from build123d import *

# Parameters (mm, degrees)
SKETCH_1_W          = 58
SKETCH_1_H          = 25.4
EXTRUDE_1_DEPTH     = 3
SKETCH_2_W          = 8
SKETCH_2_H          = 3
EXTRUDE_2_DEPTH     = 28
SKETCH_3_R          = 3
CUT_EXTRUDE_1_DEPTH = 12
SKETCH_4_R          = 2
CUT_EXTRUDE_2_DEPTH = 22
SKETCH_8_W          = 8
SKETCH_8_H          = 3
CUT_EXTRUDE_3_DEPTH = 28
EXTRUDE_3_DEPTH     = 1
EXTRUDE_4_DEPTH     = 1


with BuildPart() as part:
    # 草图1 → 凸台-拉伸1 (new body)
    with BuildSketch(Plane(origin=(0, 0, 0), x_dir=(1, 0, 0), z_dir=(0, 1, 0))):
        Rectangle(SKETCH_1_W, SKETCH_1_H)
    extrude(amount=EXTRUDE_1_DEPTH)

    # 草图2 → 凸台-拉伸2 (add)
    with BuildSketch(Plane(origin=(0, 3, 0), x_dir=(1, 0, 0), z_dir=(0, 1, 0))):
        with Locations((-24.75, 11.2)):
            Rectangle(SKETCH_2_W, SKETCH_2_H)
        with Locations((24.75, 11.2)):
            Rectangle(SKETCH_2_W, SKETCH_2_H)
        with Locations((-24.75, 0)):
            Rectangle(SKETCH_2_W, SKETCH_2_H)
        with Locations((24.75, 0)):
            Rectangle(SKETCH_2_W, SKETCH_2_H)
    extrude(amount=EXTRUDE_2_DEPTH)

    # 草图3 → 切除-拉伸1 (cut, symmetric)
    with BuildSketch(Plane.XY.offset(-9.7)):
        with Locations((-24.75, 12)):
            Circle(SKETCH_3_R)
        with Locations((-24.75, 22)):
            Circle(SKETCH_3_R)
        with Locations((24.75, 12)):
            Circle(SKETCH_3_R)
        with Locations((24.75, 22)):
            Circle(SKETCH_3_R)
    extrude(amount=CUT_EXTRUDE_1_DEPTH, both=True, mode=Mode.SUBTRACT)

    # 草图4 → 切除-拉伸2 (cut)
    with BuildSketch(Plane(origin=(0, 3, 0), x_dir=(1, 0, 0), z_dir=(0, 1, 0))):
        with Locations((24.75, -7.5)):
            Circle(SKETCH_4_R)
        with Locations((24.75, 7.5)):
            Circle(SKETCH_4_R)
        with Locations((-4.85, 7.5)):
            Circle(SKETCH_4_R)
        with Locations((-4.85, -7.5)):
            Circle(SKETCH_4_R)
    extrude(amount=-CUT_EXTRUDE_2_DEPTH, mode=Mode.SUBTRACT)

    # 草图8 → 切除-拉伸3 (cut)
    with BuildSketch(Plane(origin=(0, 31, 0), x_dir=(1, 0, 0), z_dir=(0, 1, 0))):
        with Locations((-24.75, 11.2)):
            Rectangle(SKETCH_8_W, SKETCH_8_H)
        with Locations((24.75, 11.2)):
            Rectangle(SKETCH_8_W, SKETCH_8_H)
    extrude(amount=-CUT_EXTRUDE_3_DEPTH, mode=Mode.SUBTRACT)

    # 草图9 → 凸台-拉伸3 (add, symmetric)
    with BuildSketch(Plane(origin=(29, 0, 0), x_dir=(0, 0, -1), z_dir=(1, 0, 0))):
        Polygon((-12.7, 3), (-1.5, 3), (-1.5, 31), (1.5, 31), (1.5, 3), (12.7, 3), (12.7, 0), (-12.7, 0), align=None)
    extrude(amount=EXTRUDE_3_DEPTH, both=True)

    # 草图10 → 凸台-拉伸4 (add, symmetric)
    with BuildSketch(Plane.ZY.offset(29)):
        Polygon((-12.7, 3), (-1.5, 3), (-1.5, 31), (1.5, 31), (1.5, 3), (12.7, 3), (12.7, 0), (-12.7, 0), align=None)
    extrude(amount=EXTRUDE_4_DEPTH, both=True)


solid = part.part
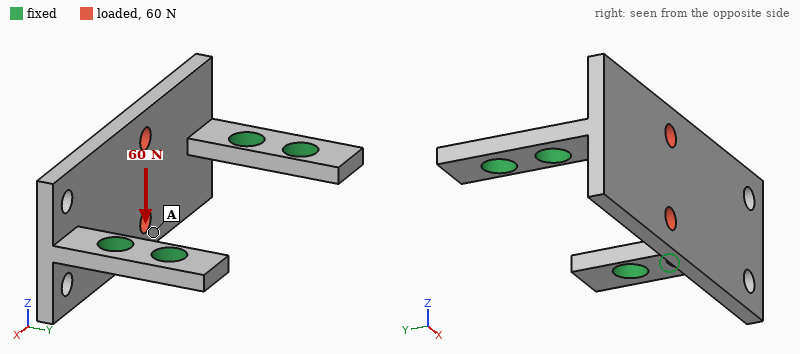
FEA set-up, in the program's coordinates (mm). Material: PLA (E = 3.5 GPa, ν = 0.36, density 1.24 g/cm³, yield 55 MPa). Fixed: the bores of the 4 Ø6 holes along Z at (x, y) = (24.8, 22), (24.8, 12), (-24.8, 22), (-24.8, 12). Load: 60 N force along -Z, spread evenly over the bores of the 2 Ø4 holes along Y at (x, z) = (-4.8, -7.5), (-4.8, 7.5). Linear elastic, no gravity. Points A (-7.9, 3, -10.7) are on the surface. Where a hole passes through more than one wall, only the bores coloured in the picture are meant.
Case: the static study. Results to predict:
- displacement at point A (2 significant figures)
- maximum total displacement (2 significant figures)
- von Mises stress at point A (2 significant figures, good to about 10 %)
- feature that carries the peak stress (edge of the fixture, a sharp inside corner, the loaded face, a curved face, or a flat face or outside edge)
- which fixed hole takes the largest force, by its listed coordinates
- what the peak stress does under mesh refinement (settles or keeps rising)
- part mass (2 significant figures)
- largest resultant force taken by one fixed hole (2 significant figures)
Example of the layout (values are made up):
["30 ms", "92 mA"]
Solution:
["0.16 mm", "0.21 mm", "2.3 MPa", "edge of the fixture", "(-24.8, 12)", "keeps rising", "7.0 g", "36 N"]
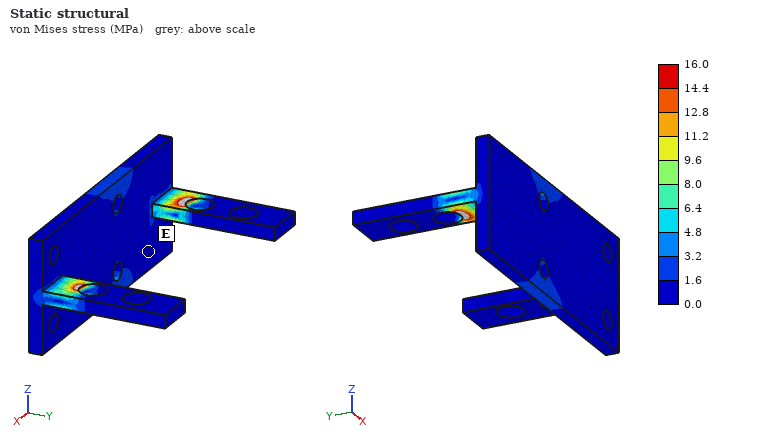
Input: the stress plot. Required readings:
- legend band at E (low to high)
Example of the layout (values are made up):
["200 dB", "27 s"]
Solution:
["0.0 to 1.6 MPa"]
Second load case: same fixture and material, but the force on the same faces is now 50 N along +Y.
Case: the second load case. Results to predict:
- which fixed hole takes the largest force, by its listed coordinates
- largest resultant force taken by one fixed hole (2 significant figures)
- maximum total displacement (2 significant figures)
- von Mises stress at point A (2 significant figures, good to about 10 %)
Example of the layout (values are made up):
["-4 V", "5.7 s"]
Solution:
["(-24.8, 12)", "43 N", "0.20 mm", "5.5 MPa"]
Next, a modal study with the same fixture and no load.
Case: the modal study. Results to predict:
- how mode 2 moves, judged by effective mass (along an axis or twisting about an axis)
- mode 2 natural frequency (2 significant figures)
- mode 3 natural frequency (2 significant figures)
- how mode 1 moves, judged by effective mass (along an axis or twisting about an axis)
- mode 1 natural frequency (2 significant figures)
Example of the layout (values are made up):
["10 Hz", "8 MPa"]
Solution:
["along Y", "1900 Hz", "2200 Hz", "along Z", "1000 Hz"]
